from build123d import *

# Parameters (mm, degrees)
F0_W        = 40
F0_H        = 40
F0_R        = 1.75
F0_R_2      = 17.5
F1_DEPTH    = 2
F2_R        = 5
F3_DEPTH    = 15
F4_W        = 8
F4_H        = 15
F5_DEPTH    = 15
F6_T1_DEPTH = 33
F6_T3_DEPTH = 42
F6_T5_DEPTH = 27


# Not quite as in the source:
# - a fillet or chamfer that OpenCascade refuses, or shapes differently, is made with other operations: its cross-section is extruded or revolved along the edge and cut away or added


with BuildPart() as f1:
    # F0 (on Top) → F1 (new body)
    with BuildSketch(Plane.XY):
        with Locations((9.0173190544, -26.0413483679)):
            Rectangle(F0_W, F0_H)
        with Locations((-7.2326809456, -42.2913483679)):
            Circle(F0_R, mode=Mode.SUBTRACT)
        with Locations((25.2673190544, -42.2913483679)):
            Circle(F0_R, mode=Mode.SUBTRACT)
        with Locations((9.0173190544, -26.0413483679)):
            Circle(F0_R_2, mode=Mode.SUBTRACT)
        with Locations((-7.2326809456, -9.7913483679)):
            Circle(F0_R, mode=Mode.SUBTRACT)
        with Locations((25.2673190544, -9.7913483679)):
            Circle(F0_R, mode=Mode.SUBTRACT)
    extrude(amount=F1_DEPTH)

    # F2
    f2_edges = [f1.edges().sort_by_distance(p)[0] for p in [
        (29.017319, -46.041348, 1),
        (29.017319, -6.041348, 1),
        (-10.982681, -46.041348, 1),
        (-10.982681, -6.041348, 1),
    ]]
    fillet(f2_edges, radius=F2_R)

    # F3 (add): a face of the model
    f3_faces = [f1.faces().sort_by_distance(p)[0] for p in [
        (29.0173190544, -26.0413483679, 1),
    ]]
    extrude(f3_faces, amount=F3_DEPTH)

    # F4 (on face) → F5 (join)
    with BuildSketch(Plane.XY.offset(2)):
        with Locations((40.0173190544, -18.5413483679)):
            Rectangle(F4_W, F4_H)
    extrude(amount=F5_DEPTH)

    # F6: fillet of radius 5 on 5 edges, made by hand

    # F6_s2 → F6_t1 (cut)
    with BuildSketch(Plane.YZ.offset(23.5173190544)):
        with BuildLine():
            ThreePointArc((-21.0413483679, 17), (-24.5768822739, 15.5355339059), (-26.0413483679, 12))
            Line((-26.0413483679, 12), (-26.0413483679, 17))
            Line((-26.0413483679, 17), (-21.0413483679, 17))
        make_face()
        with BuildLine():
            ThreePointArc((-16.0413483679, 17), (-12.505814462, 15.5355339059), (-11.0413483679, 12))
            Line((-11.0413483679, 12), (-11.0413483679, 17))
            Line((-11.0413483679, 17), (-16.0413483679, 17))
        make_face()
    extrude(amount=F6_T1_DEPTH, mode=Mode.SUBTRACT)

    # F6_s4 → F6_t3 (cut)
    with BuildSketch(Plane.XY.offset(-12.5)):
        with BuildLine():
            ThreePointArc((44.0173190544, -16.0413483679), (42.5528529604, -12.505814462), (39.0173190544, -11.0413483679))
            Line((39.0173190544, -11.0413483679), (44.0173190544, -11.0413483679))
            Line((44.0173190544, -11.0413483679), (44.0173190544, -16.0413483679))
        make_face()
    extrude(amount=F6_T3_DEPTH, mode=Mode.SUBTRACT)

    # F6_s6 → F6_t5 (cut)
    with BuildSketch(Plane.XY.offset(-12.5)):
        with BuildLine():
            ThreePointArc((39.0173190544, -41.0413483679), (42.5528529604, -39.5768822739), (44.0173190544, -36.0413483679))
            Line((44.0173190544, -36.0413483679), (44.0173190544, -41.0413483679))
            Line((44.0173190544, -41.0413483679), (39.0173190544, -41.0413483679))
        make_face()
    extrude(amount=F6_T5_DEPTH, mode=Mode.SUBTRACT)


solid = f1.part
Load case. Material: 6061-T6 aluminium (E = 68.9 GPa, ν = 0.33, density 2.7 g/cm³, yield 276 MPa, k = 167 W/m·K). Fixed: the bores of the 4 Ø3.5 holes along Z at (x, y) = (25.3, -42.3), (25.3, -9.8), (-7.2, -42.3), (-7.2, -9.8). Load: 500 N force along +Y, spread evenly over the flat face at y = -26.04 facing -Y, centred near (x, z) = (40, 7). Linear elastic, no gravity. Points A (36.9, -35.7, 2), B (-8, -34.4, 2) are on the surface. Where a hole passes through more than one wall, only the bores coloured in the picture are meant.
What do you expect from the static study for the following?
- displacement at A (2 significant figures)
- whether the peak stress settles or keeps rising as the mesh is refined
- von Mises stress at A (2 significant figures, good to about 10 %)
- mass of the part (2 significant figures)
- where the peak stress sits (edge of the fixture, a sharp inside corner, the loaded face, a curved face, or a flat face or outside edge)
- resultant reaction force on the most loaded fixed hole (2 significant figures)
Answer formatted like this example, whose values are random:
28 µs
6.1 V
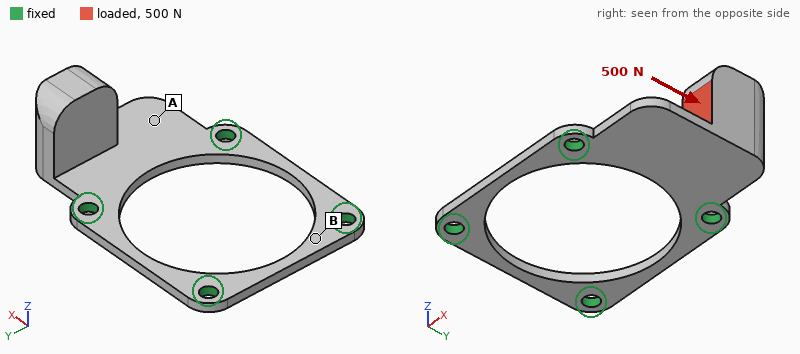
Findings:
0.074 mm
keeps rising
46 MPa
9.9 g
edge of the fixture
380 N
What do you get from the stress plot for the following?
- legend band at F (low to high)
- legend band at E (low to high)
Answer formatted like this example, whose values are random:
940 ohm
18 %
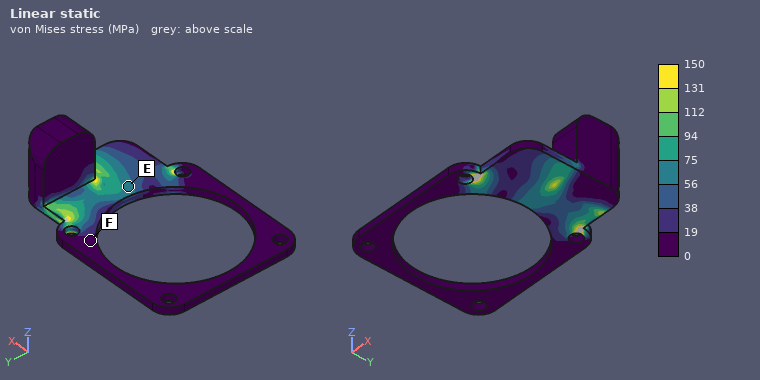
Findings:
0 to 19 MPa
56 to 75 MPa
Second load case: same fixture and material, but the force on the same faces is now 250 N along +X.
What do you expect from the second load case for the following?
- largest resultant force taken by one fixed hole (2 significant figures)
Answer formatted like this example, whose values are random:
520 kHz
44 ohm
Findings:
160 N
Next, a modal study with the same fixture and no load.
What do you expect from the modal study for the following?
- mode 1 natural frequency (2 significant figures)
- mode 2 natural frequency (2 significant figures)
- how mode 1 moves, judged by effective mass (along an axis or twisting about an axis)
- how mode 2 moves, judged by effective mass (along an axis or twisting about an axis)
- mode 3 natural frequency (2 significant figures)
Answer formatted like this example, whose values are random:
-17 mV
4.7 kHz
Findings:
1400 Hz
3800 Hz
along Z
along Y
5800 Hz
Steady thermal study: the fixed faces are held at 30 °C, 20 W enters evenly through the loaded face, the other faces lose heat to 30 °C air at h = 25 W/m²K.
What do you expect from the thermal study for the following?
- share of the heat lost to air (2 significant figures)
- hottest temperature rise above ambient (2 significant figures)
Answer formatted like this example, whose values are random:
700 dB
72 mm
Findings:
8.2 %
55 K
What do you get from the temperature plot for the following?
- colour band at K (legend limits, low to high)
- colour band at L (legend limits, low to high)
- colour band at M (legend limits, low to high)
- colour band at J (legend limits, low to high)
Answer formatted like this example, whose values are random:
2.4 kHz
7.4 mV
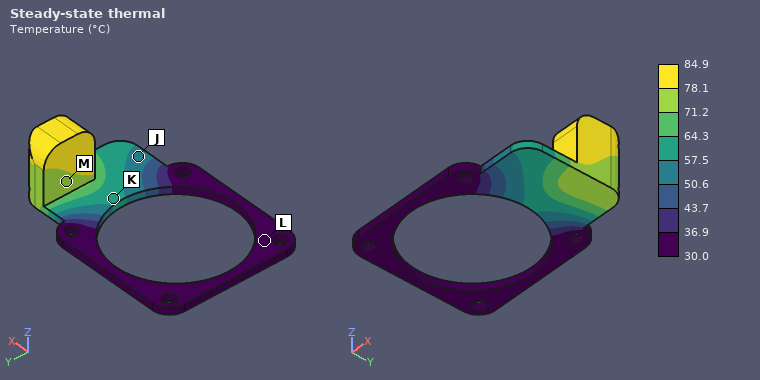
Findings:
57.5 to 64.3 °C
30.0 to 36.9 °C
71.2 to 78.1 °C
50.6 to 57.5 °C
